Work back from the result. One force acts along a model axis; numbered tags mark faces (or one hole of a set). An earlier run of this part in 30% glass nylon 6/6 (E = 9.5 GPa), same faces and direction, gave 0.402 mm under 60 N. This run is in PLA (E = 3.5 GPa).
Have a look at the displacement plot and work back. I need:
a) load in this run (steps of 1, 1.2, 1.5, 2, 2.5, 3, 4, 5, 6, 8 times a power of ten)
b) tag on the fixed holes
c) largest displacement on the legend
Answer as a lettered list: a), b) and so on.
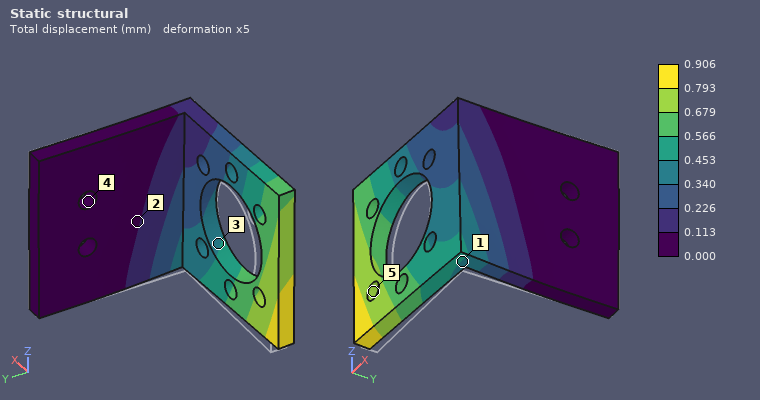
a) 50 N
b) 4
c) 0.906 mm
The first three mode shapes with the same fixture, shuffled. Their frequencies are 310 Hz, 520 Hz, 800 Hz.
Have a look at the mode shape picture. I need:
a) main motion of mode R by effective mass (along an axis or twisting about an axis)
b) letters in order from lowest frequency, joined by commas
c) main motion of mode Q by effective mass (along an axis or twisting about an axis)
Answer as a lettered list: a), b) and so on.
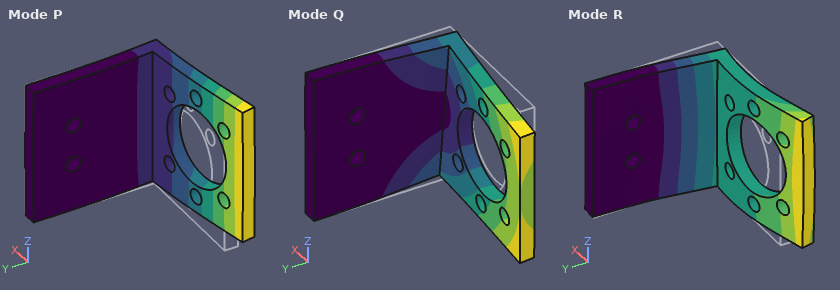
a) along X
b) P, Q, R
c) along Z
